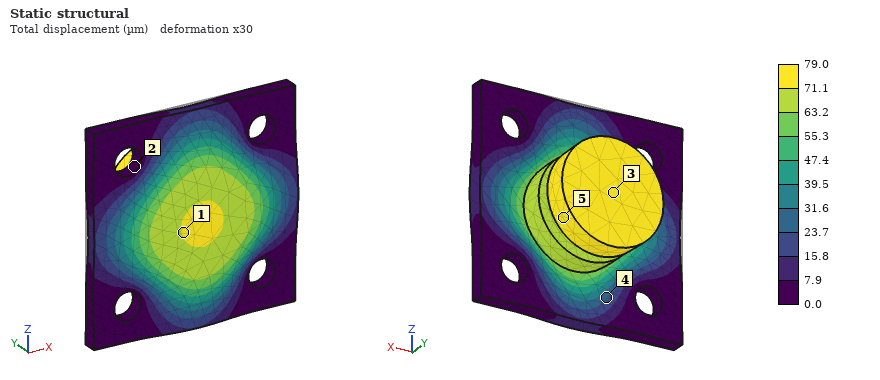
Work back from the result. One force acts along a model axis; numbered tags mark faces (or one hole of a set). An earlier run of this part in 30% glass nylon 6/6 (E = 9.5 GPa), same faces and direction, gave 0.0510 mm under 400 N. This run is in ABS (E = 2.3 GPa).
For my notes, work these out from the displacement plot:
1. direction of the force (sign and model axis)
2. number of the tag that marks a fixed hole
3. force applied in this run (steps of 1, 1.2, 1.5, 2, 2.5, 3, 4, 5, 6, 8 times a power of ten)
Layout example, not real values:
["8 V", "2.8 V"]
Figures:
["-Y", "2", "150 N"]
